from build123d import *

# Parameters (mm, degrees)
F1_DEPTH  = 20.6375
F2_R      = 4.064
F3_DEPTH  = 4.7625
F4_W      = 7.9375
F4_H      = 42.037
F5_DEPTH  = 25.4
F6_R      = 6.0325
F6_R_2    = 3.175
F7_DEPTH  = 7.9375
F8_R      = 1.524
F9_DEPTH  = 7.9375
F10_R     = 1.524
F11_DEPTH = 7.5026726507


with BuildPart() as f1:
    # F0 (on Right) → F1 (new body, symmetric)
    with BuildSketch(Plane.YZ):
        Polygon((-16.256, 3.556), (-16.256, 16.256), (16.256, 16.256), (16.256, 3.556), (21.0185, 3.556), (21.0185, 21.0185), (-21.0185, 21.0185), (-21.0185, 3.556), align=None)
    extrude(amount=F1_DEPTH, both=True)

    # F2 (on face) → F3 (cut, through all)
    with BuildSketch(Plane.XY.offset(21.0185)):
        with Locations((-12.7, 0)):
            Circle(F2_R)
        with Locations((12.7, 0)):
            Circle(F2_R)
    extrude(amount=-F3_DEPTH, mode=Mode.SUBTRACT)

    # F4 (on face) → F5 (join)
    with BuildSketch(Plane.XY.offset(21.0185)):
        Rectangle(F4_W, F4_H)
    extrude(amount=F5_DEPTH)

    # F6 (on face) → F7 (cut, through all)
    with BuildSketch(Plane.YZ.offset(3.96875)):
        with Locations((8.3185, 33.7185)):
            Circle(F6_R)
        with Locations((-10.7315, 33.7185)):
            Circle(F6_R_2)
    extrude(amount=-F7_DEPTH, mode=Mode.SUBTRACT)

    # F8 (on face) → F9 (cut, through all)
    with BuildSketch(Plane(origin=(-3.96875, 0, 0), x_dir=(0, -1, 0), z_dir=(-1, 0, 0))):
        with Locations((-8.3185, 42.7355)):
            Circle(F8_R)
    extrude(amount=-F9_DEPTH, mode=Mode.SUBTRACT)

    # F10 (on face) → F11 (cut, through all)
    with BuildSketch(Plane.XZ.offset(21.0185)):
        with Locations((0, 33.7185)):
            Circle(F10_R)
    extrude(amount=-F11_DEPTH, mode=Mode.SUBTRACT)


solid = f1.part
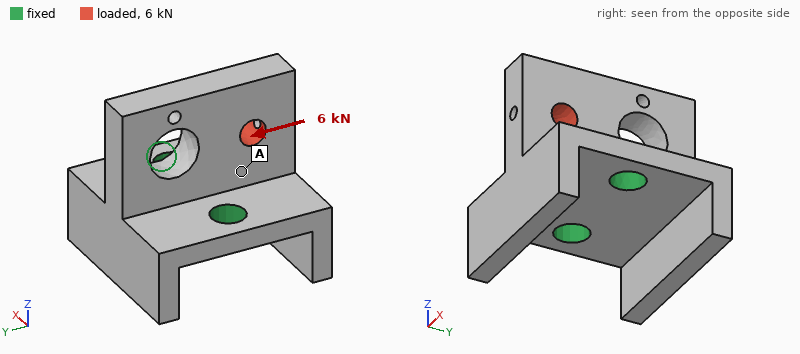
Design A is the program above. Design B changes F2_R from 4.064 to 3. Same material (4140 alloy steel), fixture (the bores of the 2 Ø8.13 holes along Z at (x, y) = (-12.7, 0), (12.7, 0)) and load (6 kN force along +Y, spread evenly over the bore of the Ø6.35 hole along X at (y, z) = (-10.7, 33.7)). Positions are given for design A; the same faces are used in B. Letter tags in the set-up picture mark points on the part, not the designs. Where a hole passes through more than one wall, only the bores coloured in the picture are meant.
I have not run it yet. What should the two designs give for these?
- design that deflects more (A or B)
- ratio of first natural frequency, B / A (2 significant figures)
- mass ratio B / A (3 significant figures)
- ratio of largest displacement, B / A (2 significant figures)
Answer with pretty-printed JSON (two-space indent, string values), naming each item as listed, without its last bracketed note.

{
  "design that deflects more": "B",
  "ratio of first natural frequency, B / A": "0.85",
  "mass ratio B / A": "1.01",
  "ratio of largest displacement, B / A": "1.4"
}
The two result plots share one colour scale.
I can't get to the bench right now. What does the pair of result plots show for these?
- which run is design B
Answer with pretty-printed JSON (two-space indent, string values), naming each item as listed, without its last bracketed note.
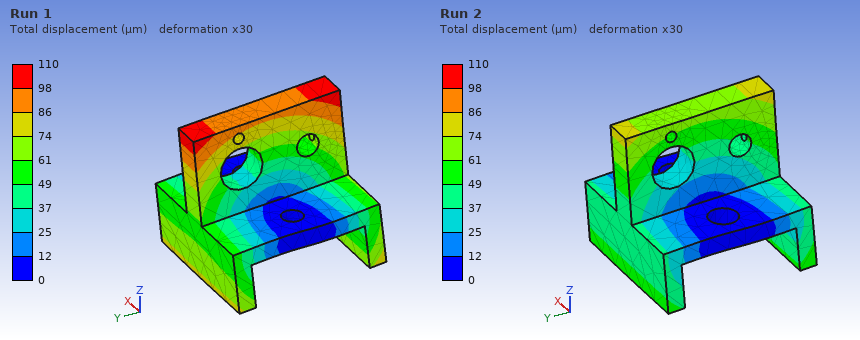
{
  "which run is design B": "Run 1"
}
